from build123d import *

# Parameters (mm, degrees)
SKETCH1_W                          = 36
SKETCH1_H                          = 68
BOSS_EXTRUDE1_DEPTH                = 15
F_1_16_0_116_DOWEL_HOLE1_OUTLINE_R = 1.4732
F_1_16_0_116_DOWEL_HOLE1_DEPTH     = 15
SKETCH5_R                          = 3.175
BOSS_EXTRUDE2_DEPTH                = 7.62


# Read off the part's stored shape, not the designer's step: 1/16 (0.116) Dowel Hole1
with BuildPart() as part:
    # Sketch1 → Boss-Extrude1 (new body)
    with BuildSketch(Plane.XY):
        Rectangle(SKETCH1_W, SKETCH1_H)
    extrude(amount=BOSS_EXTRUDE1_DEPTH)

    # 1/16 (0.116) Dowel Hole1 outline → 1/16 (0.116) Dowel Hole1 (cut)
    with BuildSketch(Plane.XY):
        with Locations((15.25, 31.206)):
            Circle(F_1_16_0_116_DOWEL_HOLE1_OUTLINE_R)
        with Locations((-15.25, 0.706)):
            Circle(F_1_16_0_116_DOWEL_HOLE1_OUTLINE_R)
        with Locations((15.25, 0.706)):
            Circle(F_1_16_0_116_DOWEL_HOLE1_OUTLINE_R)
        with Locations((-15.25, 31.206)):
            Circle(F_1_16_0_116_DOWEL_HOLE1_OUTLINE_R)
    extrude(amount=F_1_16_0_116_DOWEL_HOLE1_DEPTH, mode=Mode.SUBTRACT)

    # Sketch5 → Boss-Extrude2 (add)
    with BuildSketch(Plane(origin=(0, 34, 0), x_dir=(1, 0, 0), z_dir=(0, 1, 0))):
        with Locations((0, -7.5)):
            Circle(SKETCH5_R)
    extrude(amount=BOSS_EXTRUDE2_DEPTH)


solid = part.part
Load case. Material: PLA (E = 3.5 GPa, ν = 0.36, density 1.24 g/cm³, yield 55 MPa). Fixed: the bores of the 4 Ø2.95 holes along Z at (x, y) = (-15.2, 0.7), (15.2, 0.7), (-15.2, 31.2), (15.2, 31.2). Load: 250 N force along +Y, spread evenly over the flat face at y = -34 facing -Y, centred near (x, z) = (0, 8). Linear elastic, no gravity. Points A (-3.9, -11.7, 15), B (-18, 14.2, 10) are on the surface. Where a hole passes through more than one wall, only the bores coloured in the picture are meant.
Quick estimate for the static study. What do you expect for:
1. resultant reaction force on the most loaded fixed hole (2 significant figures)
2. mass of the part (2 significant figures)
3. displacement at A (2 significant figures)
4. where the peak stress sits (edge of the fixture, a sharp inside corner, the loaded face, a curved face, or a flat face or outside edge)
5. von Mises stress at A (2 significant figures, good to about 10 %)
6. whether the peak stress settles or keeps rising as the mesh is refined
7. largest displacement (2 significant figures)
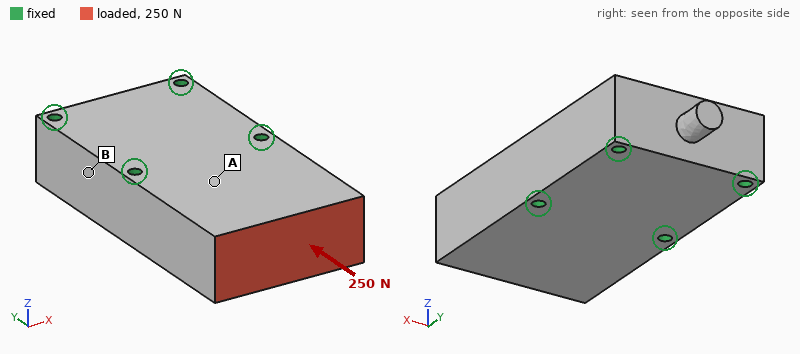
110 N
45 g
2.6 µm
edge of the fixture
0.36 MPa
keeps rising
5.4 µm
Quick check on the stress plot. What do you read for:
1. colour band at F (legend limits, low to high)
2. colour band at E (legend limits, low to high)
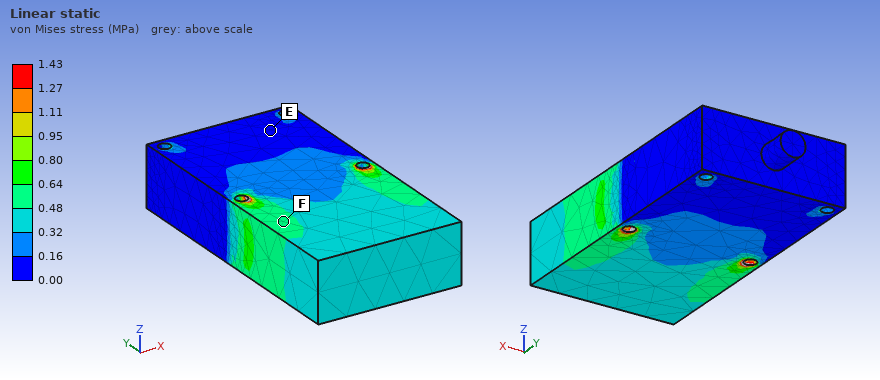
0.48 to 0.64 MPa
0.00 to 0.16 MPa
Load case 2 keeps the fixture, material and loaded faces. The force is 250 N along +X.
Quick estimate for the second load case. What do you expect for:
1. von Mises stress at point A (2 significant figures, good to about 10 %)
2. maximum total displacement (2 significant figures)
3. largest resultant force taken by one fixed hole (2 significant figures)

1.1 MPa
37 µm
300 N
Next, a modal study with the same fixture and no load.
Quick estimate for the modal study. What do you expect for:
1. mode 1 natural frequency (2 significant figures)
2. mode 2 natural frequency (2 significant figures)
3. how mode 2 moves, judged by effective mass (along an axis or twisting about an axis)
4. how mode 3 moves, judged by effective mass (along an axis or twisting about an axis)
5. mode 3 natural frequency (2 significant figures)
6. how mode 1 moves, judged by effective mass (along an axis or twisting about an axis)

2600 Hz
5000 Hz
along X
twisting about Y
5400 Hz
along Z
